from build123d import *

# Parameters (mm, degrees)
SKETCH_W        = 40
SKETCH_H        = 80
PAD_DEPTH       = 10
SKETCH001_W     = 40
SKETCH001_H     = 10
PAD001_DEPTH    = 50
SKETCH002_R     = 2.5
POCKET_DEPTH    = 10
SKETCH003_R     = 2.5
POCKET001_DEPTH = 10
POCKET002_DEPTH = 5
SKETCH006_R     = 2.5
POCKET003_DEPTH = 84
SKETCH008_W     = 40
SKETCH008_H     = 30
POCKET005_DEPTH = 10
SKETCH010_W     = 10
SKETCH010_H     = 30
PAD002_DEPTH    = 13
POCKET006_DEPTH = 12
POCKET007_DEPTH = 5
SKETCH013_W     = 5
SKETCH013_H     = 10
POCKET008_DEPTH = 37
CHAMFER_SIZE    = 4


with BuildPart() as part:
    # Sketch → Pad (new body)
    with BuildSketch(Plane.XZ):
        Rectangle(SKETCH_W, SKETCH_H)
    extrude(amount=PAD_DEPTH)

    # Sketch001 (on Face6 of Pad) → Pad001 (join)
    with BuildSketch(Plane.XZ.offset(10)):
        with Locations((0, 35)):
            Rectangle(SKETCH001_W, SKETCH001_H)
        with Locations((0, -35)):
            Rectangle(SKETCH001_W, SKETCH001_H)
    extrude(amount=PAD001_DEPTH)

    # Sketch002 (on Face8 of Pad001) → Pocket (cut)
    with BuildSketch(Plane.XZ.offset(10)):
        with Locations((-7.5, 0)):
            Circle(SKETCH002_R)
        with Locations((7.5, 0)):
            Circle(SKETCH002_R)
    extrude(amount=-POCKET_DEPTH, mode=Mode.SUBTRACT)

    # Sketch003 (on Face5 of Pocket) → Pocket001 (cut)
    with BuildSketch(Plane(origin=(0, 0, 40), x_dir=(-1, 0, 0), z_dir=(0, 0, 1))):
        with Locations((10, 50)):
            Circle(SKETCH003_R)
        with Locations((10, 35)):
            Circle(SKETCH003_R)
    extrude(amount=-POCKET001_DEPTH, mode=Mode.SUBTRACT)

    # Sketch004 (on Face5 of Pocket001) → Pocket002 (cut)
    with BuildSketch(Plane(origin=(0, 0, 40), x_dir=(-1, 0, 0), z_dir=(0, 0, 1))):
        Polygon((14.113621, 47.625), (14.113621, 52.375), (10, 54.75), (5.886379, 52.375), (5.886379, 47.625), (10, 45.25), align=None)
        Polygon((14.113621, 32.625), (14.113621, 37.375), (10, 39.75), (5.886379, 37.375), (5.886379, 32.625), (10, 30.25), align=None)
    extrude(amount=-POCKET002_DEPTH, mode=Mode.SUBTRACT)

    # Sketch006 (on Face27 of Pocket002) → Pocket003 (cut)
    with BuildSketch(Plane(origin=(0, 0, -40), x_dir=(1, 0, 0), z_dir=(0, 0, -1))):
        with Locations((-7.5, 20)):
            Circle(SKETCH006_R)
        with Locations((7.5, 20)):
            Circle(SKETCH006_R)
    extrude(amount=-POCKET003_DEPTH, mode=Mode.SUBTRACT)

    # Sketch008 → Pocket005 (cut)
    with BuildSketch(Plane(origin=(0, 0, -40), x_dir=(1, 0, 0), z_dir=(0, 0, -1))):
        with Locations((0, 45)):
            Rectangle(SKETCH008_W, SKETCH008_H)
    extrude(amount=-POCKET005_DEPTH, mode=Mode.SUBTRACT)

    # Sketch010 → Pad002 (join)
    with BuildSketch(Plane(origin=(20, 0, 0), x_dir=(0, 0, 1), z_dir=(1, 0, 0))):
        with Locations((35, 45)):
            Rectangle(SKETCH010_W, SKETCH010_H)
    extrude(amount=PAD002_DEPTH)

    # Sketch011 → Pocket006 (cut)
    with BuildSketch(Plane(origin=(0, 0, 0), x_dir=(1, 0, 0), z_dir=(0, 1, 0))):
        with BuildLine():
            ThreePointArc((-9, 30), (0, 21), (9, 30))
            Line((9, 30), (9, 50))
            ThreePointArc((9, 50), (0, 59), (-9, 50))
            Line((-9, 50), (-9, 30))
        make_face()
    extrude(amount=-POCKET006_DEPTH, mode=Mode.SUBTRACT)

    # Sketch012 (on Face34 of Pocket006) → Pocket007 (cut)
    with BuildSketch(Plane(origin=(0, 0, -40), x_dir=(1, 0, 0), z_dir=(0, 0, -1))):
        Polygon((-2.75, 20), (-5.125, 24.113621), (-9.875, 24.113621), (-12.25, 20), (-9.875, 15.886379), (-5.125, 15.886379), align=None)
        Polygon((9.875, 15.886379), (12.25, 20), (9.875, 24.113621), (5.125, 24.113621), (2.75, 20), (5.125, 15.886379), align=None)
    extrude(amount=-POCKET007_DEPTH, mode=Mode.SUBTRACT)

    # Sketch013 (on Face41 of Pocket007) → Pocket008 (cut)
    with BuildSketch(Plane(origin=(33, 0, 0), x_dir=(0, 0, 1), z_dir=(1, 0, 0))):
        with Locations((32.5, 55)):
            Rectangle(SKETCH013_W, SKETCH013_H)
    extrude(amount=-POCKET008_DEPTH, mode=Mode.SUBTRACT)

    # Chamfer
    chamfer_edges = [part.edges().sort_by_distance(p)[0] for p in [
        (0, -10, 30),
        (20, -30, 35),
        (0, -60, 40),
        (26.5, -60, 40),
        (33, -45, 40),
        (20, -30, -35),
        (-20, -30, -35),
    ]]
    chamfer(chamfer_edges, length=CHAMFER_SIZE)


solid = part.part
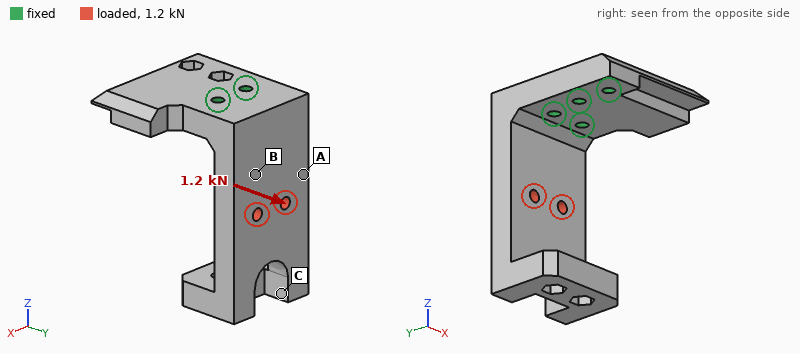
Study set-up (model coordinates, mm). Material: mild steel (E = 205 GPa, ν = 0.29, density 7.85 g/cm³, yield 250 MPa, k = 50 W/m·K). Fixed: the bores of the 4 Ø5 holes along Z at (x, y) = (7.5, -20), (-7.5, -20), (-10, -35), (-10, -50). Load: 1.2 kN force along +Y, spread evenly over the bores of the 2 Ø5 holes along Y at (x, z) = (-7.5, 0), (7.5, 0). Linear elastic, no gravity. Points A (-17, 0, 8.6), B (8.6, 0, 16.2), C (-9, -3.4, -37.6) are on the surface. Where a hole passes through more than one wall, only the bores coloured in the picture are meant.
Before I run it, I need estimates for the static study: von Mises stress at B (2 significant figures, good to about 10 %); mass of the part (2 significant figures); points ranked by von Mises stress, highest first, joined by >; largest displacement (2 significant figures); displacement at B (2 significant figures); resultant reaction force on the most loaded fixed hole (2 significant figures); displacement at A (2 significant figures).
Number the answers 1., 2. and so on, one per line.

1. 28 MPa
2. 440 g
3. B > A > C
4. 0.10 mm
5. 0.022 mm
6. 660 N
7. 0.031 mm
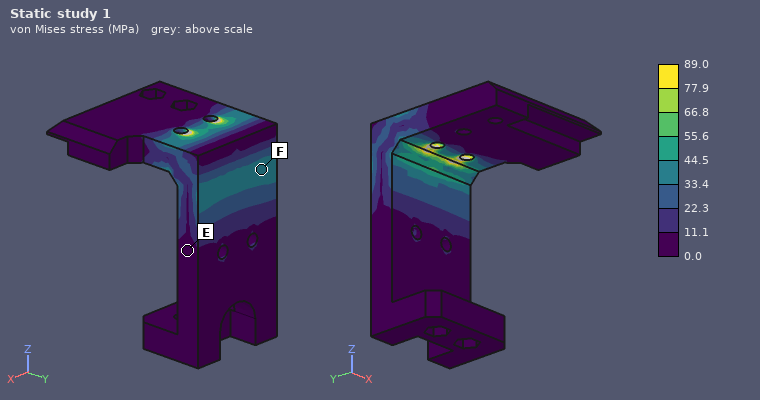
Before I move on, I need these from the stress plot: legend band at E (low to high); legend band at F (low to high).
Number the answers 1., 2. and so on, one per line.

1. 0.0 to 11.1 MPa
2. 33.4 to 44.5 MPa
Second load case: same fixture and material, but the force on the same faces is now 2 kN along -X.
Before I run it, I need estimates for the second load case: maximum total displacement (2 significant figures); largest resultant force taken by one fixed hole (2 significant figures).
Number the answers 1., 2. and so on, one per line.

1. 48 µm
2. 3.2 kN
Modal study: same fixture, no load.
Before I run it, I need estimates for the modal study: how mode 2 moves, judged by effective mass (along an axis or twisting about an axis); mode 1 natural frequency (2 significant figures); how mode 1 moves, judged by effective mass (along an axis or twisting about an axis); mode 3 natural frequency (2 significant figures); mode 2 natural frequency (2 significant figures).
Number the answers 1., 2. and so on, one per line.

1. along X
2. 1000 Hz
3. along Y
4. 3800 Hz
5. 2000 Hz
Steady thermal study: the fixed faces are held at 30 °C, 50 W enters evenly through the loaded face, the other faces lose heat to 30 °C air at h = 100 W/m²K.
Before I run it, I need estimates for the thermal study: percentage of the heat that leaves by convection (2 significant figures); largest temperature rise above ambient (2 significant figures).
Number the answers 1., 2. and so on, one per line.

1. 61 %
2. 57 K
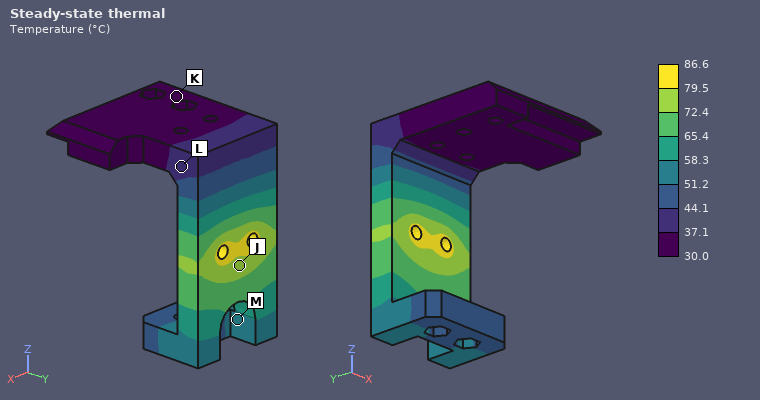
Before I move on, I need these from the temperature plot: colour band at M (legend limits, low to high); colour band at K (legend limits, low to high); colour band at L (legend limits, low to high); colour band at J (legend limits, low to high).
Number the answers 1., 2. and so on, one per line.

1. 51.2 to 58.3 °C
2. 30.0 to 37.1 °C
3. 37.1 to 44.1 °C
4. 72.4 to 79.5 °C
